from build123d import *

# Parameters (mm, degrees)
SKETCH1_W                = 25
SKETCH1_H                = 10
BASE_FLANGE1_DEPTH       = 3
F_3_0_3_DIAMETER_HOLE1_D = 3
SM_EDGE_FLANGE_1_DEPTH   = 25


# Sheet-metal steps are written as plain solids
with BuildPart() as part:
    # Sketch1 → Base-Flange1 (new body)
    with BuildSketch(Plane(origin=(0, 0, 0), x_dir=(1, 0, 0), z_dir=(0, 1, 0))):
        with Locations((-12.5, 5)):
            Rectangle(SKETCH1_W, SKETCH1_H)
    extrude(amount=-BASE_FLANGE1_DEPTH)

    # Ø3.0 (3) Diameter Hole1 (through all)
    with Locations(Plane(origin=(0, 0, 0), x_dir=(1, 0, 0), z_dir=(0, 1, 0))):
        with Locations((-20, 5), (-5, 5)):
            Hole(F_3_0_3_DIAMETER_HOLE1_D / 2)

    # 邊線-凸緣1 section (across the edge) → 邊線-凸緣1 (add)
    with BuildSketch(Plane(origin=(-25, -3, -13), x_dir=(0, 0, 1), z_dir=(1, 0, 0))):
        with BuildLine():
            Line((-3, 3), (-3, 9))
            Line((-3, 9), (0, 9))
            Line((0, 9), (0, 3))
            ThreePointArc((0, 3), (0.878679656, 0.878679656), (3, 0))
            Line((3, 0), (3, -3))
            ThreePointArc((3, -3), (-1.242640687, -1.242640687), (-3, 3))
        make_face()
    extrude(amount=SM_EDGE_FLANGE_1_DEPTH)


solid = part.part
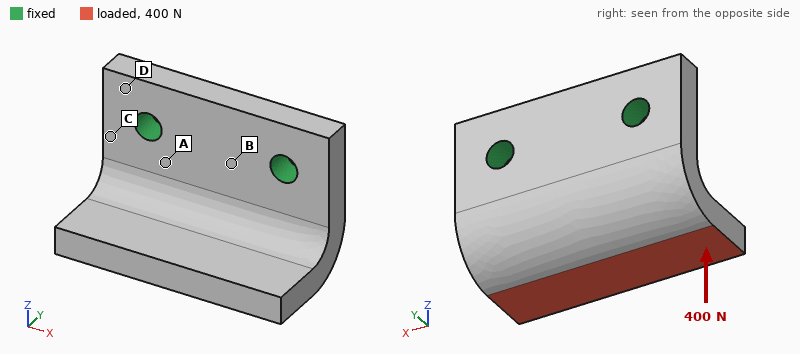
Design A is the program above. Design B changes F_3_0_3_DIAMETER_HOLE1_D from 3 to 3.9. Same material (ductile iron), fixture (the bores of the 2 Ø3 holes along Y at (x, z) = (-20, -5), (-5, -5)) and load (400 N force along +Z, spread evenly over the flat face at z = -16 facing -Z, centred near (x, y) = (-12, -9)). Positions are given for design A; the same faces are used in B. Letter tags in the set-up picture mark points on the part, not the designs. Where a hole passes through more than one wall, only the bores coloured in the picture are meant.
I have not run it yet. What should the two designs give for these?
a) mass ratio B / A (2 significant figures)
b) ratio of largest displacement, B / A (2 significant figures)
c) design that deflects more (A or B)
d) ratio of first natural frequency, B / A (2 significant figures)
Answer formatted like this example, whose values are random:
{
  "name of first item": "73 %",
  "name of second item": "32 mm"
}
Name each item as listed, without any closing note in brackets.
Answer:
{
  "mass ratio B / A": "0.98",
  "ratio of largest displacement, B / A": "0.92",
  "design that deflects more": "A",
  "ratio of first natural frequency, B / A": "1.1"
}
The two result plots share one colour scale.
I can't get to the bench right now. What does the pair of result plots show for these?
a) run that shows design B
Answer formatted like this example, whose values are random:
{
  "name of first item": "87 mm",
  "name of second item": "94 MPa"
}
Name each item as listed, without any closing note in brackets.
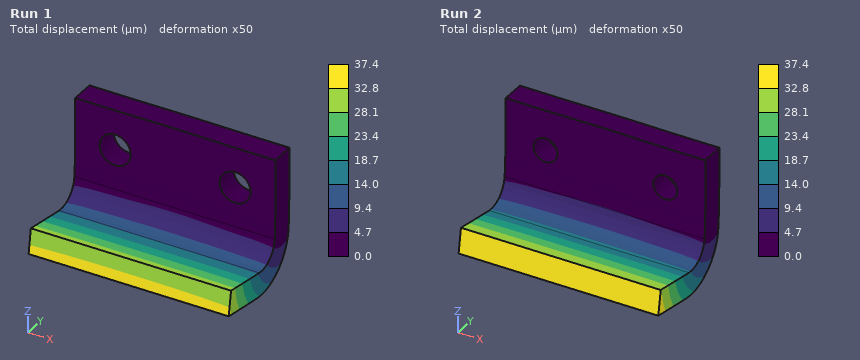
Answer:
{
  "run that shows design B": "Run 1"
}
